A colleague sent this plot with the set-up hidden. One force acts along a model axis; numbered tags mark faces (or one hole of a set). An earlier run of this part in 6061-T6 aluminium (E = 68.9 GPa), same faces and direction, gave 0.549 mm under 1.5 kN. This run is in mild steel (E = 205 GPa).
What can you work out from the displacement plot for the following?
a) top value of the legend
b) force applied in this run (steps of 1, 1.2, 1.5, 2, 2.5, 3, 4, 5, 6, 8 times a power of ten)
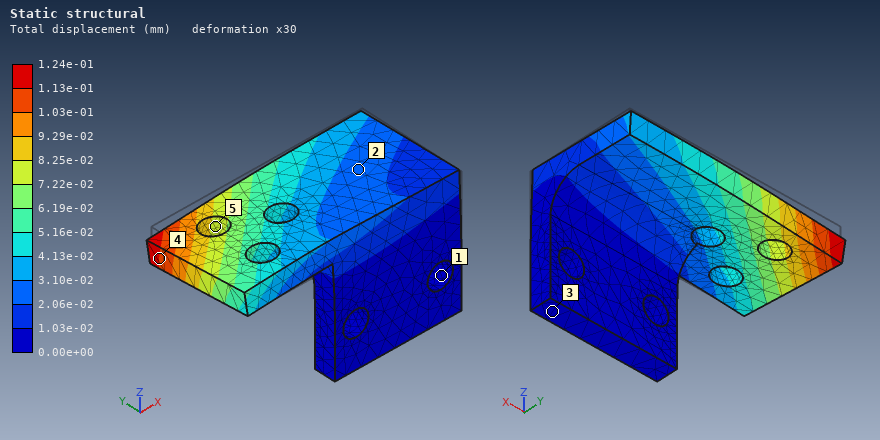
1.24e-01 mm
1 kN
